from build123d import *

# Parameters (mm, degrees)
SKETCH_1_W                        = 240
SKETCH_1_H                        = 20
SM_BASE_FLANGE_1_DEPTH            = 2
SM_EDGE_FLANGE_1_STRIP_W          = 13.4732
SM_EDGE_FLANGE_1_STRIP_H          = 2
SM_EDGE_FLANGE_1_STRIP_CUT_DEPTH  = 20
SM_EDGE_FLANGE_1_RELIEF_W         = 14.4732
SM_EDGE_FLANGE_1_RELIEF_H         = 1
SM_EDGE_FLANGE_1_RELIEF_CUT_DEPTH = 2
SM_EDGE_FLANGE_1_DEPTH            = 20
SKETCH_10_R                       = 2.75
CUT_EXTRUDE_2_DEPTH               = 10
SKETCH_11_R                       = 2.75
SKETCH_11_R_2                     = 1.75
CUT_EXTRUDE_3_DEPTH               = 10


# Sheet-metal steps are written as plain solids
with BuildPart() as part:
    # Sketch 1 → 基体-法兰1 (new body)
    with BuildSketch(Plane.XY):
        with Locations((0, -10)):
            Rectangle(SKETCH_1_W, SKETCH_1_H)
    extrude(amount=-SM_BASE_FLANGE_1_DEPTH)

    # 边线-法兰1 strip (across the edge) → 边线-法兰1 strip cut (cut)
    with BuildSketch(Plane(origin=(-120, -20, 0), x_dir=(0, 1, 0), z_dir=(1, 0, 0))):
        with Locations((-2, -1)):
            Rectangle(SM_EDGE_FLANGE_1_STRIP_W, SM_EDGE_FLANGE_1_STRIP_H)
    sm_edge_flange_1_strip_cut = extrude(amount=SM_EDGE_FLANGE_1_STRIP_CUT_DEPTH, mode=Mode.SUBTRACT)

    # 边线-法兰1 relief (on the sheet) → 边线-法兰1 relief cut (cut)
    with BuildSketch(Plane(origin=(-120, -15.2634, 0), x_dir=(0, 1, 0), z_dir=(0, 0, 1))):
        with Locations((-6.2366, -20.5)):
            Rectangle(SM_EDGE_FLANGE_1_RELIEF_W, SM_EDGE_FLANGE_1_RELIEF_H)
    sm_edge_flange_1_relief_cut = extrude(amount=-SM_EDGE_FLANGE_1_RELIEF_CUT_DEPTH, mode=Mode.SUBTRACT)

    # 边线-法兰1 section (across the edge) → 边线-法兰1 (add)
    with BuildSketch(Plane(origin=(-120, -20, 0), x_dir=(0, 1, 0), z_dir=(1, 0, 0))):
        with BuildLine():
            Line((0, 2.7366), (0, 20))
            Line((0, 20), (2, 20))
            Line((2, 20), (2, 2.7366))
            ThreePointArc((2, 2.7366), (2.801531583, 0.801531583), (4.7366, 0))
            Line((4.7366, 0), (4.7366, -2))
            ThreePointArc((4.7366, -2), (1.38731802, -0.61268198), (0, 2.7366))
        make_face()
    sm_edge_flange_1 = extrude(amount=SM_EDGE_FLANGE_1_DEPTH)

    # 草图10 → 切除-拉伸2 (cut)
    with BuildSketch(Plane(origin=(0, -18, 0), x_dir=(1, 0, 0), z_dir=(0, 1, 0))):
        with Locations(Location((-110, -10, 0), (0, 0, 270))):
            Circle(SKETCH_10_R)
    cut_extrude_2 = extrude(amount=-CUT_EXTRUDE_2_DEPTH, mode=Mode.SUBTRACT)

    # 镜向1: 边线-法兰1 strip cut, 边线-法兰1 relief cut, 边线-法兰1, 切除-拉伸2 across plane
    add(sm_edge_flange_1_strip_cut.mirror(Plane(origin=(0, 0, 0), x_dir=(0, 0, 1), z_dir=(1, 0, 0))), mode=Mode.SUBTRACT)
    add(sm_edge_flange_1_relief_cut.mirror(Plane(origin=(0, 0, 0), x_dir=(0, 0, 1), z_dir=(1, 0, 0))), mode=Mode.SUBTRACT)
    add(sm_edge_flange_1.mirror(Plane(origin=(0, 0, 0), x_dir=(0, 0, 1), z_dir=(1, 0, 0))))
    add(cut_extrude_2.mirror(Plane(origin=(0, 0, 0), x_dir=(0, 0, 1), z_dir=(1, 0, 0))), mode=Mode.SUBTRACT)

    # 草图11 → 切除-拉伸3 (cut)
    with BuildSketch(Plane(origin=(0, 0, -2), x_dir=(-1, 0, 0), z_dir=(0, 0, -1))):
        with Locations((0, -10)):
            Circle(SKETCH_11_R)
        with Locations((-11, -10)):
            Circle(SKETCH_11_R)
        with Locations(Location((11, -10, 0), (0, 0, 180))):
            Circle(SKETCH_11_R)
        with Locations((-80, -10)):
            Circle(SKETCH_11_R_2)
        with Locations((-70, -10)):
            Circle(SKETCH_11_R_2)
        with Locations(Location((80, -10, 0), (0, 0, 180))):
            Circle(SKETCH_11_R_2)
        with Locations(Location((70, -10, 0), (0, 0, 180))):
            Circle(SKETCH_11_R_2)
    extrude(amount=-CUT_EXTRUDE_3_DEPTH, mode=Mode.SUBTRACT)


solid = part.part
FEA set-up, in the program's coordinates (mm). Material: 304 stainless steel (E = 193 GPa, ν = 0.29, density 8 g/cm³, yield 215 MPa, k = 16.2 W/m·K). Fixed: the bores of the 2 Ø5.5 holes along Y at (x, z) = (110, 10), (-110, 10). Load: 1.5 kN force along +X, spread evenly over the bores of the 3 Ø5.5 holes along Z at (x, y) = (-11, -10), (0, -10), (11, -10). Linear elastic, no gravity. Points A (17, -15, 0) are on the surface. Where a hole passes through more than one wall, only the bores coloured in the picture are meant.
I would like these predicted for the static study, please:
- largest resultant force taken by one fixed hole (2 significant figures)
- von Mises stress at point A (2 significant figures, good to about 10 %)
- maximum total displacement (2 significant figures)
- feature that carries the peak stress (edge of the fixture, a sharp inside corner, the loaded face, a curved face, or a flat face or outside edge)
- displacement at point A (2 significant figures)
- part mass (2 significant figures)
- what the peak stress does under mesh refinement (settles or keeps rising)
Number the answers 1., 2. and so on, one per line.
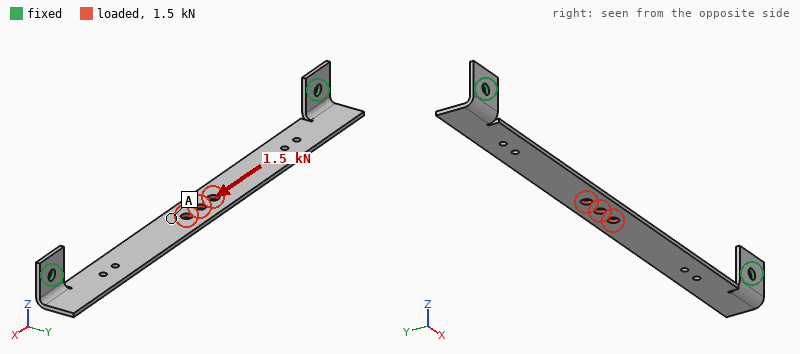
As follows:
1. 750 N
2. 26 MPa
3. 42 µm
4. a sharp inside corner
5. 36 µm
6. 86 g
7. keeps rising
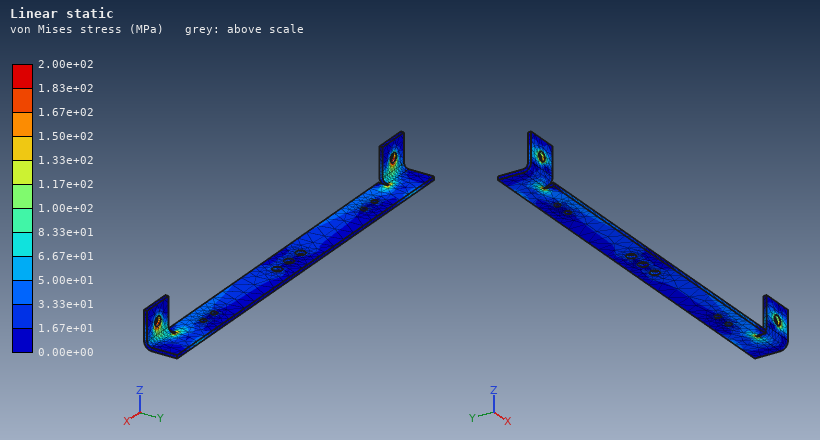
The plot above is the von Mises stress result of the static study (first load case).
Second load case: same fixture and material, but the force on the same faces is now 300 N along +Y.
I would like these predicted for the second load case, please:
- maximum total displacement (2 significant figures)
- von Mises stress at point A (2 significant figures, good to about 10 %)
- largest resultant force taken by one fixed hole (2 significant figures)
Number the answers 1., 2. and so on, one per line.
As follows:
1. 0.21 mm
2. 21 MPa
3. 420 N
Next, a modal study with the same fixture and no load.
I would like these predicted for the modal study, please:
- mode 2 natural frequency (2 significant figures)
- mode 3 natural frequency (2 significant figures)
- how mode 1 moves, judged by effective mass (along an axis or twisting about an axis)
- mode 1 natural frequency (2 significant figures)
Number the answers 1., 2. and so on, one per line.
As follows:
1. 570 Hz
2. 940 Hz
3. along Z
4. 200 Hz
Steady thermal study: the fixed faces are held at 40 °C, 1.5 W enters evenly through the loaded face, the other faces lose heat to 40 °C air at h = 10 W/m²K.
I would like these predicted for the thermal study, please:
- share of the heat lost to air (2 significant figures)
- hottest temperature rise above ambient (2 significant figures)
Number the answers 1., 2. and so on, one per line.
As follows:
1. 93 %
2. 40 K
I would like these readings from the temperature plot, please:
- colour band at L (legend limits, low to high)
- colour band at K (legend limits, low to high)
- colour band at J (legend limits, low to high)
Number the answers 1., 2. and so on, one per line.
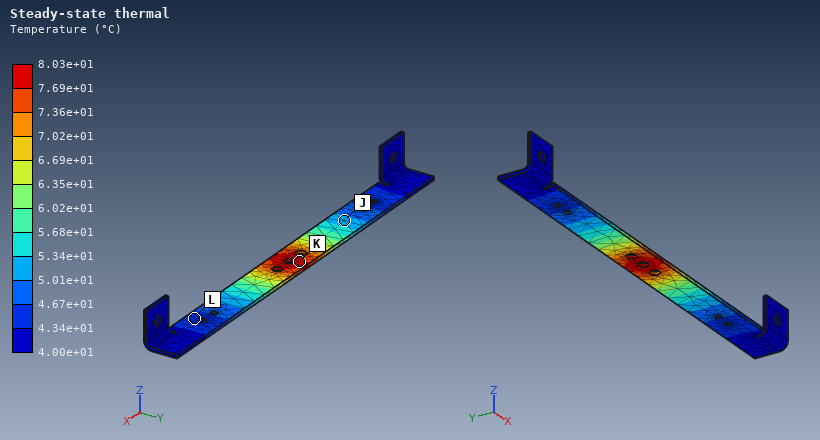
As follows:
1. 4.34e+01 to 4.67e+01 °C
2. 7.69e+01 to 8.03e+01 °C
3. 5.01e+01 to 5.34e+01 °C
